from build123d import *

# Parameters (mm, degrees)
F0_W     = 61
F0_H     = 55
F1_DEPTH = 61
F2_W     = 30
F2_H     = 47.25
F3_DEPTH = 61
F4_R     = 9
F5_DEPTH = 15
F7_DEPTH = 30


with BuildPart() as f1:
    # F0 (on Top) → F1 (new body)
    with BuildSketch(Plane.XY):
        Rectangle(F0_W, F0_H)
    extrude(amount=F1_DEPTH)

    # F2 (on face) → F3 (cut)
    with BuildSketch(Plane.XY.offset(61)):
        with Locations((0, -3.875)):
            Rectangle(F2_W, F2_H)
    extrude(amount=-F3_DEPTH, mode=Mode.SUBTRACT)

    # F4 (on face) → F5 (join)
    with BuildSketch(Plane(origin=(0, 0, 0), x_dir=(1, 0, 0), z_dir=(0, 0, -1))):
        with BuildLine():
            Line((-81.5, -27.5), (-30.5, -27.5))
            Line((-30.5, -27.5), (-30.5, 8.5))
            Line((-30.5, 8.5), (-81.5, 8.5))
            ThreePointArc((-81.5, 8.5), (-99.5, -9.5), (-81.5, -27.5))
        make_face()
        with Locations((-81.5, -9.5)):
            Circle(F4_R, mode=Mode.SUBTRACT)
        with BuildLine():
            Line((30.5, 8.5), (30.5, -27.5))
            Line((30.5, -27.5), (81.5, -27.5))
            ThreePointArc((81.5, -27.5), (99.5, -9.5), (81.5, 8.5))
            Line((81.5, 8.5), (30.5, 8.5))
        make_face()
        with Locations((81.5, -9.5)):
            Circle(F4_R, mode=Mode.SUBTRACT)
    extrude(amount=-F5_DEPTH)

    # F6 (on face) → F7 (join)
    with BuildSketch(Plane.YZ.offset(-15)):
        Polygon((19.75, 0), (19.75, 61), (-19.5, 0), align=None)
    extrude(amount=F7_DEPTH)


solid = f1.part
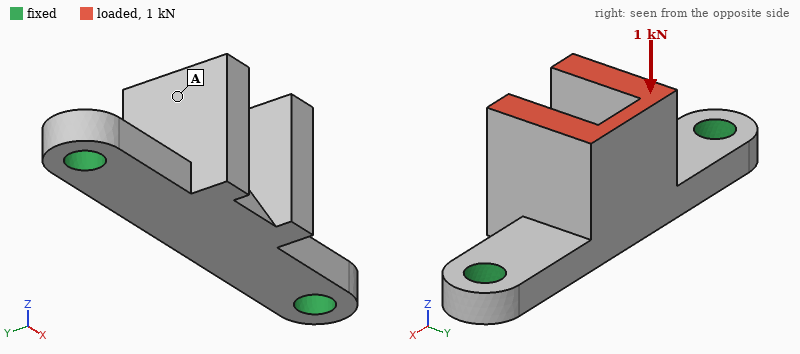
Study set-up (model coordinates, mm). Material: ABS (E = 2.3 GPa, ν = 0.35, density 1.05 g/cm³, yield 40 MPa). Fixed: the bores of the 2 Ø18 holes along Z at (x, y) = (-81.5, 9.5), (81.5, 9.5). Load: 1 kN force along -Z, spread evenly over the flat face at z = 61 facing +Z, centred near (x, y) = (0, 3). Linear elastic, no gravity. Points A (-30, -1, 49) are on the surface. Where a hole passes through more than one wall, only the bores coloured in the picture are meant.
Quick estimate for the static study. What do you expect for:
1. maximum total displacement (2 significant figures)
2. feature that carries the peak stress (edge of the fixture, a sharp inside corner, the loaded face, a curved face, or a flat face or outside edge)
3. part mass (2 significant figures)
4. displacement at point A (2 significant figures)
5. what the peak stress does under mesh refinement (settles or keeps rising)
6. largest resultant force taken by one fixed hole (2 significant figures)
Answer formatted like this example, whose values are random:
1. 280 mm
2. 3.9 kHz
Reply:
1. 0.61 mm
2. edge of the fixture
3. 230 g
4. 0.45 mm
5. keeps rising
6. 550 N
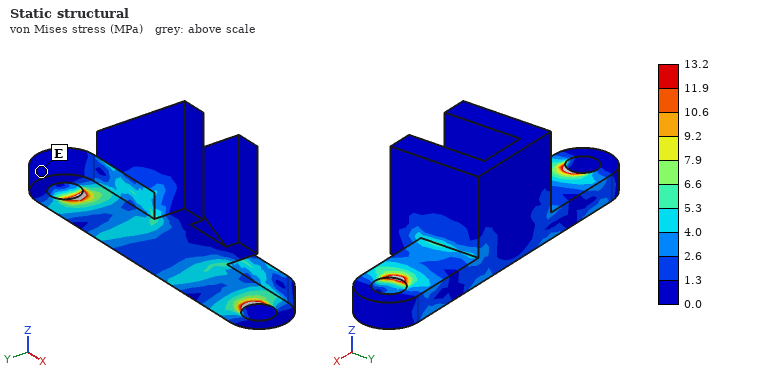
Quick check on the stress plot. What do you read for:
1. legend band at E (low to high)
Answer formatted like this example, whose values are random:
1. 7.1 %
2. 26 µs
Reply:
1. 0.0 to 1.3 MPa
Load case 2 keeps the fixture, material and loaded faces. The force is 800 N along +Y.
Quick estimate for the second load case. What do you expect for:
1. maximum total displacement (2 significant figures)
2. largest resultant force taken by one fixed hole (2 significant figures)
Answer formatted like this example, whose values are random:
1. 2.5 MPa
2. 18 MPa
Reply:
1. 2.5 mm
2. 410 N
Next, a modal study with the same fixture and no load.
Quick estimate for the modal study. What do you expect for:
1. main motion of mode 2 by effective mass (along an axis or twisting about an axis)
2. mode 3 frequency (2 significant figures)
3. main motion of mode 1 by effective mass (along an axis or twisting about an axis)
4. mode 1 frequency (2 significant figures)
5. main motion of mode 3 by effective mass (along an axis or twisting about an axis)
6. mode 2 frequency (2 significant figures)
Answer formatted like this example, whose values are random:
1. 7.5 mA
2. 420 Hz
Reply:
1. along Z
2. 1000 Hz
3. along Y
4. 400 Hz
5. along X
6. 680 Hz
